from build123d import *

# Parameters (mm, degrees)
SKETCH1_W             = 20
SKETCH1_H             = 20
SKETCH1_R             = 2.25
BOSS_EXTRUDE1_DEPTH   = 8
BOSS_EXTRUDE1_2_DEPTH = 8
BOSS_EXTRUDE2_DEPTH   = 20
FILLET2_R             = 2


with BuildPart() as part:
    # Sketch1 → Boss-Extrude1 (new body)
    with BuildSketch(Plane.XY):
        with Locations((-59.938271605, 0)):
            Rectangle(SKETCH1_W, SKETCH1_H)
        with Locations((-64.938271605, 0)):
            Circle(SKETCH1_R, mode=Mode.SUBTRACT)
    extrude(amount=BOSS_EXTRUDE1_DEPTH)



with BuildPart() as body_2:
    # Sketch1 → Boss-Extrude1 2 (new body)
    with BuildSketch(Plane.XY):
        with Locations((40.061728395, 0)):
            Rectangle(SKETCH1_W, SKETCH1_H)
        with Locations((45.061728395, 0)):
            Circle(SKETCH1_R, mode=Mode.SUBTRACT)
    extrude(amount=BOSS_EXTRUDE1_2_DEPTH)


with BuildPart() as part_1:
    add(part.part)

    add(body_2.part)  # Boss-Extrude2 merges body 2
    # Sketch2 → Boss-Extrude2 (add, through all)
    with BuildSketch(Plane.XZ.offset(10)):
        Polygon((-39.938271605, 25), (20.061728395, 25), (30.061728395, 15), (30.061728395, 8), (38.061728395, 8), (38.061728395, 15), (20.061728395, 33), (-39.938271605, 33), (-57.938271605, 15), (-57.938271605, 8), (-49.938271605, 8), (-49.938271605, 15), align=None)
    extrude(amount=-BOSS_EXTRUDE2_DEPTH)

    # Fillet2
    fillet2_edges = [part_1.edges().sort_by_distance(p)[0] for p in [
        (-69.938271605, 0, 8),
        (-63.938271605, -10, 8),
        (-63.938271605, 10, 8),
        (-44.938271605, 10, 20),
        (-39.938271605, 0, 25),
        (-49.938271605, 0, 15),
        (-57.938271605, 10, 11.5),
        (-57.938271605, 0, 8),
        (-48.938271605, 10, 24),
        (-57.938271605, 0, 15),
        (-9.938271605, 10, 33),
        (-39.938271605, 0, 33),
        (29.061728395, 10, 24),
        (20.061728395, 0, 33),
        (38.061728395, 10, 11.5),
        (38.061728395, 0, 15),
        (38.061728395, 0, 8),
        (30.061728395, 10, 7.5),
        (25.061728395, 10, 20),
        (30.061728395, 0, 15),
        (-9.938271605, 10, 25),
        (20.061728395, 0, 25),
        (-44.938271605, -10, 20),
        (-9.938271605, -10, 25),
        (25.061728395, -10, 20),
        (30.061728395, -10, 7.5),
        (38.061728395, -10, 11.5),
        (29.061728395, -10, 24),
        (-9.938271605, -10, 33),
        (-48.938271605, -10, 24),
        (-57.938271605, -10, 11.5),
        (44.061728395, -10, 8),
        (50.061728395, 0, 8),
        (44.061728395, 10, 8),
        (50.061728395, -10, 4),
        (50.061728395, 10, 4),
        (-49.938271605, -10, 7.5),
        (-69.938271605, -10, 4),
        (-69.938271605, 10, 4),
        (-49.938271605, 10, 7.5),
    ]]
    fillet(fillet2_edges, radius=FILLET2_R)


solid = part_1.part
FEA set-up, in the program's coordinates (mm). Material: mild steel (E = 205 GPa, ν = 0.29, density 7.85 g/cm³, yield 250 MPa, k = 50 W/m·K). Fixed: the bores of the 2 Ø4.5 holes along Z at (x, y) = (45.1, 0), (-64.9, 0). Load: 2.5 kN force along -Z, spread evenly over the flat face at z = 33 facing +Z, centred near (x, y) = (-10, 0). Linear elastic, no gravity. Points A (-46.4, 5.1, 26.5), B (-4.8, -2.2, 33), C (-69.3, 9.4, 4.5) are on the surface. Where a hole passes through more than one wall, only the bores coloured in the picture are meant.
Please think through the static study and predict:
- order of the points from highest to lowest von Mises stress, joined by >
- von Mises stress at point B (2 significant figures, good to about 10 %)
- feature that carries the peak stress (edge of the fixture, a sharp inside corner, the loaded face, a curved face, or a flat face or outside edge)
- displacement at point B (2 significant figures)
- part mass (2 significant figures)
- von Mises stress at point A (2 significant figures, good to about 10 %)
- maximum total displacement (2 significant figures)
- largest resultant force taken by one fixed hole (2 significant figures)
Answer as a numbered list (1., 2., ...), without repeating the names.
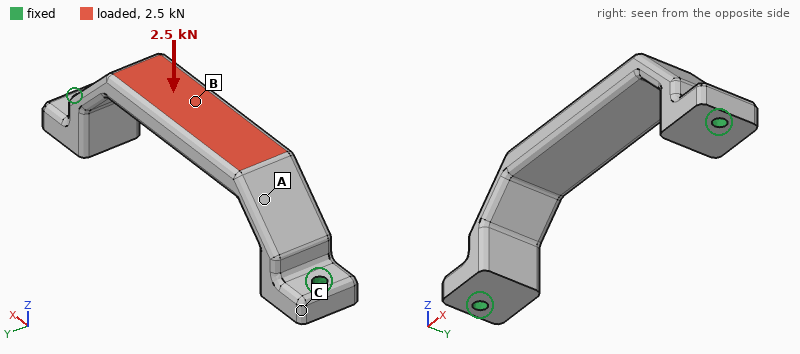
1. B > A > C
2. 68 MPa
3. a curved face
4. 33 µm
5. 170 g
6. 35 MPa
7. 36 µm
8. 1.9 kN
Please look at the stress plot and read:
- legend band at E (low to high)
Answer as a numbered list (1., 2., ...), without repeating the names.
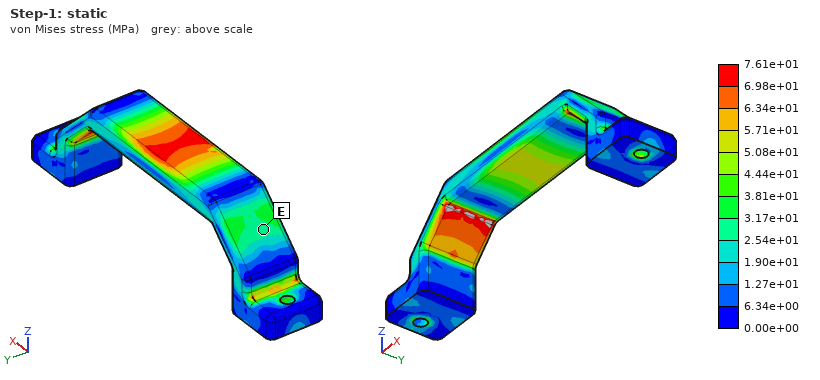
1. 2.54e+01 to 3.17e+01 MPa
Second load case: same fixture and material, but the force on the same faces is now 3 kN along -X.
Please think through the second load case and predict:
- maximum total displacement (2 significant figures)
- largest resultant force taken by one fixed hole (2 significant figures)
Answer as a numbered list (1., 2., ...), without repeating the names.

1. 34 µm
2. 1.6 kN
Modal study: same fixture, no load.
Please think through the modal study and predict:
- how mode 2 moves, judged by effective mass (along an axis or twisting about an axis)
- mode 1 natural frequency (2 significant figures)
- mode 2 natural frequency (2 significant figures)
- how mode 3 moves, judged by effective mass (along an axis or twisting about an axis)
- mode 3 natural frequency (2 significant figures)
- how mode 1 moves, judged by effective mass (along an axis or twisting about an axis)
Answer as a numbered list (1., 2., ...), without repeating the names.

1. along X
2. 3200 Hz
3. 4400 Hz
4. along Z
5. 5500 Hz
6. along Y
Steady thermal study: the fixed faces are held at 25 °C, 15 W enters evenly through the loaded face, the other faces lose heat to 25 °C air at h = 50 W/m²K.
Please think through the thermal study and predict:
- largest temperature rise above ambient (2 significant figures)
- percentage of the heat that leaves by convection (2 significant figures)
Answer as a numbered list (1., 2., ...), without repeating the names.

1. 40 K
2. 42 %
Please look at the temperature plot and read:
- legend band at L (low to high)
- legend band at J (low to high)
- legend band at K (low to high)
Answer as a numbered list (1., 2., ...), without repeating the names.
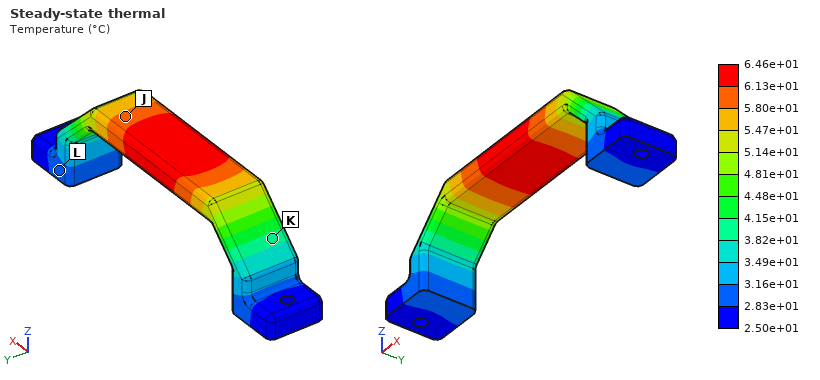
1. 2.83e+01 to 3.16e+01 °C
2. 5.80e+01 to 6.13e+01 °C
3. 3.82e+01 to 4.15e+01 °C
